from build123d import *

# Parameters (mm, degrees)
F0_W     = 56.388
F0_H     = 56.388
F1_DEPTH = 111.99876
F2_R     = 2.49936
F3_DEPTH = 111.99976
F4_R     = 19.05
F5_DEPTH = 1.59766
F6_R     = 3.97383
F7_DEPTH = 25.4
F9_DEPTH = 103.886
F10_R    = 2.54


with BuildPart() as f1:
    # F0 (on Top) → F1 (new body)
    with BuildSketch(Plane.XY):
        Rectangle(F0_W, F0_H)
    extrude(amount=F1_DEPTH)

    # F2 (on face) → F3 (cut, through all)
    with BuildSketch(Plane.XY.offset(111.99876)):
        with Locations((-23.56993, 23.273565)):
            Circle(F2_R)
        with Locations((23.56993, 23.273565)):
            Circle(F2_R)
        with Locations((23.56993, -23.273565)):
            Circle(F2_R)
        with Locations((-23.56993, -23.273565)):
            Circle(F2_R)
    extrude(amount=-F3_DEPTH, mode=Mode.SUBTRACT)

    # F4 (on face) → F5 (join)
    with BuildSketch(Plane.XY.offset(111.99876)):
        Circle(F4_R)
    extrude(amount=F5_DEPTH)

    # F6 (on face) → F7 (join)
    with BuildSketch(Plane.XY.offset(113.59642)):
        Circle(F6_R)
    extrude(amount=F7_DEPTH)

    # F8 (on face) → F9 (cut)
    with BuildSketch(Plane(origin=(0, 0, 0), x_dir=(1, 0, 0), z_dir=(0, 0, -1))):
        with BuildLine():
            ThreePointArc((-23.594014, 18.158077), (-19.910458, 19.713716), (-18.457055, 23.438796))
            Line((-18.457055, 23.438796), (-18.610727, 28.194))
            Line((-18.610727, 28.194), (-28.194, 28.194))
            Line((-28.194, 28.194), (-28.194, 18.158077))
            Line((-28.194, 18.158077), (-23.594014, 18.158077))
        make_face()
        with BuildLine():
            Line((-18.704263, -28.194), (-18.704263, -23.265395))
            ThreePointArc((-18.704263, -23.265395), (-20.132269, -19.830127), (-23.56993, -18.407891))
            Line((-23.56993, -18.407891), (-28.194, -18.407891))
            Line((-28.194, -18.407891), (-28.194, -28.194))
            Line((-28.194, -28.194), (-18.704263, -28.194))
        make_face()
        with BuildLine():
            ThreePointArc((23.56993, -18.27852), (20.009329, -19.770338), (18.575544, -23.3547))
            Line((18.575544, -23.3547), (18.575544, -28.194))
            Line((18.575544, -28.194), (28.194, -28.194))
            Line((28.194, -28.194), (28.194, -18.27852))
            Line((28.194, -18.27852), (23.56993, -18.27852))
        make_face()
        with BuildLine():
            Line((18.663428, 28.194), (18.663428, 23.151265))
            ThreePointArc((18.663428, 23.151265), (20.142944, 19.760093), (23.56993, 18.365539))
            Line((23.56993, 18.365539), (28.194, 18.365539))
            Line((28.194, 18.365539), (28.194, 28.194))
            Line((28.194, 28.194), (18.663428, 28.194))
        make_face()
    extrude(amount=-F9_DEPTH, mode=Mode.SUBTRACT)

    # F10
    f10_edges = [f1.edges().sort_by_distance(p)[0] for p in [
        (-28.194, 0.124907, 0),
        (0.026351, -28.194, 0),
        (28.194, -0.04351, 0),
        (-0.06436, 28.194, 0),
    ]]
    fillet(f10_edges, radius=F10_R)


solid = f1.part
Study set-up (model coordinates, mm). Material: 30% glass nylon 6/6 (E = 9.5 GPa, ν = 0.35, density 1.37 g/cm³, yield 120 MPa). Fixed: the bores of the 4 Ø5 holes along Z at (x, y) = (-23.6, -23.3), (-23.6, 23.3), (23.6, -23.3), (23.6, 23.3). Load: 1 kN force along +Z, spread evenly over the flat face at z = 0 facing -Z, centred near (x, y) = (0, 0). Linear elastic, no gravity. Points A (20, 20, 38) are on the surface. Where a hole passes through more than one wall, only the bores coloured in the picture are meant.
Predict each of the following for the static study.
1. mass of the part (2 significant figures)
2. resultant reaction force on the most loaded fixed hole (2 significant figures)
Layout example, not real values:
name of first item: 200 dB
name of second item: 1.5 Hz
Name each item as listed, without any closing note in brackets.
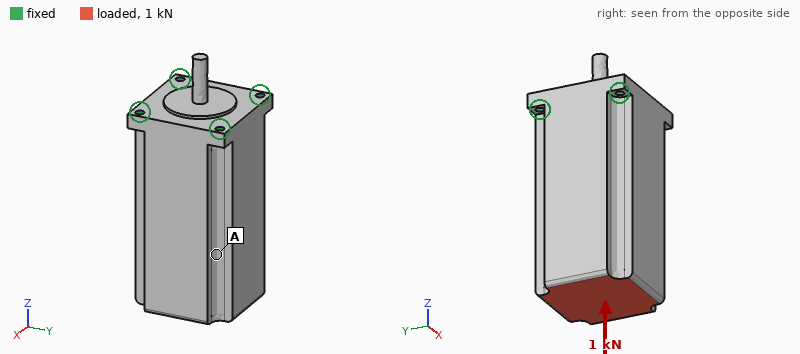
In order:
mass of the part: 440 g
resultant reaction force on the most loaded fixed hole: 270 N
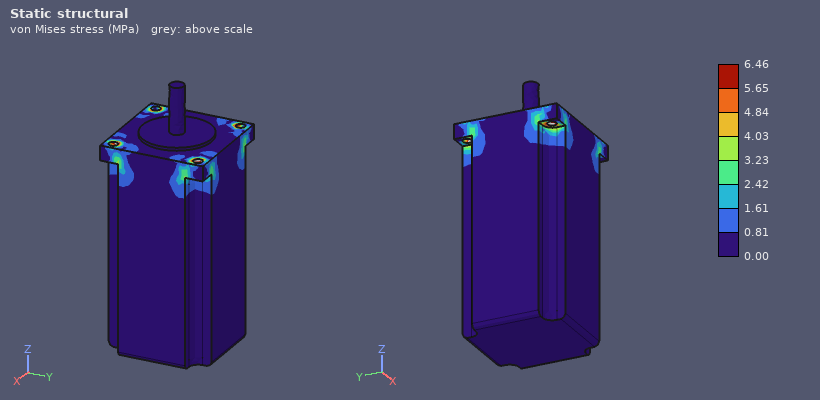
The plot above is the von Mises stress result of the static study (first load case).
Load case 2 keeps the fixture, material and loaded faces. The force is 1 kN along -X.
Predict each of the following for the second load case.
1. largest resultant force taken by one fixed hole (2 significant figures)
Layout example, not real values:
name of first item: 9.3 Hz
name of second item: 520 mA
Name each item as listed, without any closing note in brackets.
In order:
largest resultant force taken by one fixed hole: 1.3 kN
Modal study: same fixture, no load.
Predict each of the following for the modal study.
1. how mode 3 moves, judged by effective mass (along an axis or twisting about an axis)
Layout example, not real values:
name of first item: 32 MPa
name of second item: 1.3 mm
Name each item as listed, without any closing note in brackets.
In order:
how mode 3 moves, judged by effective mass: along Z
